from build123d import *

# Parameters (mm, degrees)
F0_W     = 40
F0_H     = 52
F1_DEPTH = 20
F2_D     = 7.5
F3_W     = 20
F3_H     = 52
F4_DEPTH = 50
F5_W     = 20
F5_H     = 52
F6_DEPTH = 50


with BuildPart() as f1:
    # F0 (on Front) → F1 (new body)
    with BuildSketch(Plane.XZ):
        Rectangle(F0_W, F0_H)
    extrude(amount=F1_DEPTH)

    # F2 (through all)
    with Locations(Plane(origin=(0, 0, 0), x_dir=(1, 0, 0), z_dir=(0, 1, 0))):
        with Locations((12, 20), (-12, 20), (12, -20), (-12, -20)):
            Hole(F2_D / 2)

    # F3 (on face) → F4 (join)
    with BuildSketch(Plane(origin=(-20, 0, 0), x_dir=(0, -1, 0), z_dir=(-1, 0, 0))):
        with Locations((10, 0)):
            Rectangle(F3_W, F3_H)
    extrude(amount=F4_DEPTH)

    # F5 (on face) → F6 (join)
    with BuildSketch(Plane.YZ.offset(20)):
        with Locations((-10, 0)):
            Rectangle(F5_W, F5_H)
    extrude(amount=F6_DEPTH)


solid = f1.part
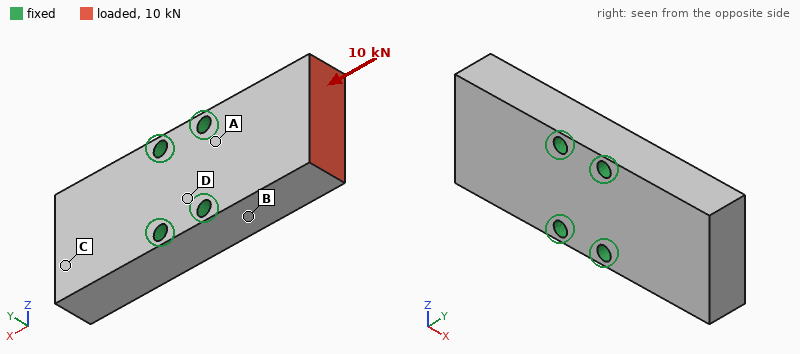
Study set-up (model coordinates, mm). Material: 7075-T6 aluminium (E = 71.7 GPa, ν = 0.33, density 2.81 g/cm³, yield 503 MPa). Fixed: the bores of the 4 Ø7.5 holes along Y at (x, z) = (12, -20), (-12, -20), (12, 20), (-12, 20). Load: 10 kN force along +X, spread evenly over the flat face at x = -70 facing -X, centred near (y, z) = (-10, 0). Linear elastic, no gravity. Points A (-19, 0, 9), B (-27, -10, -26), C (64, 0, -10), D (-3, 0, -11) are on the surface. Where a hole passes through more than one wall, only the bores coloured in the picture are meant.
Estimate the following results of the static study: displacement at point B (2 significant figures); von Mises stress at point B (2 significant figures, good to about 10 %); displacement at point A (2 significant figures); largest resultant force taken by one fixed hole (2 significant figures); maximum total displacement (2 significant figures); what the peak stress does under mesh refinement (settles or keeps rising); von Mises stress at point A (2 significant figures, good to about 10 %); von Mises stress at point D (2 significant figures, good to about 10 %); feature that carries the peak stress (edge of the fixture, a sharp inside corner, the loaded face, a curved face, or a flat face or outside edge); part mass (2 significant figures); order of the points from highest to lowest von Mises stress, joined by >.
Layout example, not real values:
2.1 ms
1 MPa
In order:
2.3 µm
11 MPa
1.8 µm
4.3 kN
8.2 µm
keeps rising
6.1 MPa
4.3 MPa
edge of the fixture
400 g
B > A > D > C
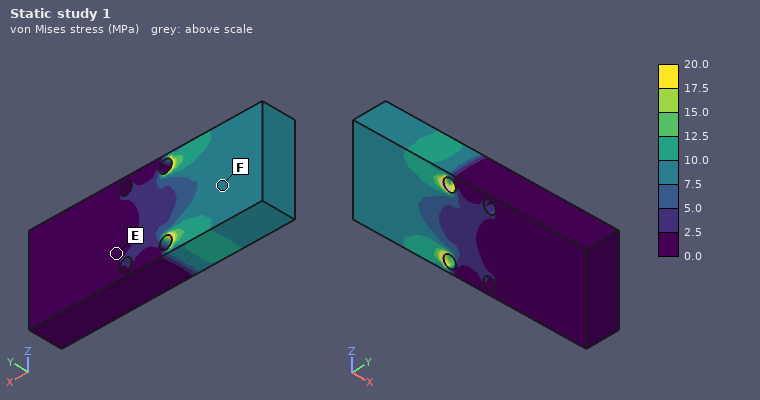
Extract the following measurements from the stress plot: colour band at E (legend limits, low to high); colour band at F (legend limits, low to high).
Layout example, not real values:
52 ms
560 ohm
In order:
0.0 to 2.5 MPa
7.5 to 10.0 MPa
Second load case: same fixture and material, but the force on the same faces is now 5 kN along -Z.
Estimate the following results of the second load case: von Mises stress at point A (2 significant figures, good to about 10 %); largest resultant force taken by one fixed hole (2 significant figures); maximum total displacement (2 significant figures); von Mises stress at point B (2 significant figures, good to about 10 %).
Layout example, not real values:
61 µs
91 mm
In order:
7.8 MPa
7.1 kN
33 µm
24 MPa
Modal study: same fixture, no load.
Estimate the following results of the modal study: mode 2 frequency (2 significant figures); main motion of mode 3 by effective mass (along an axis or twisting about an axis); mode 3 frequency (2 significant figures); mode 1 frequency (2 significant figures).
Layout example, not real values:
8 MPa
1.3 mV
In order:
4400 Hz
twisting about Y
9000 Hz
4300 Hz
